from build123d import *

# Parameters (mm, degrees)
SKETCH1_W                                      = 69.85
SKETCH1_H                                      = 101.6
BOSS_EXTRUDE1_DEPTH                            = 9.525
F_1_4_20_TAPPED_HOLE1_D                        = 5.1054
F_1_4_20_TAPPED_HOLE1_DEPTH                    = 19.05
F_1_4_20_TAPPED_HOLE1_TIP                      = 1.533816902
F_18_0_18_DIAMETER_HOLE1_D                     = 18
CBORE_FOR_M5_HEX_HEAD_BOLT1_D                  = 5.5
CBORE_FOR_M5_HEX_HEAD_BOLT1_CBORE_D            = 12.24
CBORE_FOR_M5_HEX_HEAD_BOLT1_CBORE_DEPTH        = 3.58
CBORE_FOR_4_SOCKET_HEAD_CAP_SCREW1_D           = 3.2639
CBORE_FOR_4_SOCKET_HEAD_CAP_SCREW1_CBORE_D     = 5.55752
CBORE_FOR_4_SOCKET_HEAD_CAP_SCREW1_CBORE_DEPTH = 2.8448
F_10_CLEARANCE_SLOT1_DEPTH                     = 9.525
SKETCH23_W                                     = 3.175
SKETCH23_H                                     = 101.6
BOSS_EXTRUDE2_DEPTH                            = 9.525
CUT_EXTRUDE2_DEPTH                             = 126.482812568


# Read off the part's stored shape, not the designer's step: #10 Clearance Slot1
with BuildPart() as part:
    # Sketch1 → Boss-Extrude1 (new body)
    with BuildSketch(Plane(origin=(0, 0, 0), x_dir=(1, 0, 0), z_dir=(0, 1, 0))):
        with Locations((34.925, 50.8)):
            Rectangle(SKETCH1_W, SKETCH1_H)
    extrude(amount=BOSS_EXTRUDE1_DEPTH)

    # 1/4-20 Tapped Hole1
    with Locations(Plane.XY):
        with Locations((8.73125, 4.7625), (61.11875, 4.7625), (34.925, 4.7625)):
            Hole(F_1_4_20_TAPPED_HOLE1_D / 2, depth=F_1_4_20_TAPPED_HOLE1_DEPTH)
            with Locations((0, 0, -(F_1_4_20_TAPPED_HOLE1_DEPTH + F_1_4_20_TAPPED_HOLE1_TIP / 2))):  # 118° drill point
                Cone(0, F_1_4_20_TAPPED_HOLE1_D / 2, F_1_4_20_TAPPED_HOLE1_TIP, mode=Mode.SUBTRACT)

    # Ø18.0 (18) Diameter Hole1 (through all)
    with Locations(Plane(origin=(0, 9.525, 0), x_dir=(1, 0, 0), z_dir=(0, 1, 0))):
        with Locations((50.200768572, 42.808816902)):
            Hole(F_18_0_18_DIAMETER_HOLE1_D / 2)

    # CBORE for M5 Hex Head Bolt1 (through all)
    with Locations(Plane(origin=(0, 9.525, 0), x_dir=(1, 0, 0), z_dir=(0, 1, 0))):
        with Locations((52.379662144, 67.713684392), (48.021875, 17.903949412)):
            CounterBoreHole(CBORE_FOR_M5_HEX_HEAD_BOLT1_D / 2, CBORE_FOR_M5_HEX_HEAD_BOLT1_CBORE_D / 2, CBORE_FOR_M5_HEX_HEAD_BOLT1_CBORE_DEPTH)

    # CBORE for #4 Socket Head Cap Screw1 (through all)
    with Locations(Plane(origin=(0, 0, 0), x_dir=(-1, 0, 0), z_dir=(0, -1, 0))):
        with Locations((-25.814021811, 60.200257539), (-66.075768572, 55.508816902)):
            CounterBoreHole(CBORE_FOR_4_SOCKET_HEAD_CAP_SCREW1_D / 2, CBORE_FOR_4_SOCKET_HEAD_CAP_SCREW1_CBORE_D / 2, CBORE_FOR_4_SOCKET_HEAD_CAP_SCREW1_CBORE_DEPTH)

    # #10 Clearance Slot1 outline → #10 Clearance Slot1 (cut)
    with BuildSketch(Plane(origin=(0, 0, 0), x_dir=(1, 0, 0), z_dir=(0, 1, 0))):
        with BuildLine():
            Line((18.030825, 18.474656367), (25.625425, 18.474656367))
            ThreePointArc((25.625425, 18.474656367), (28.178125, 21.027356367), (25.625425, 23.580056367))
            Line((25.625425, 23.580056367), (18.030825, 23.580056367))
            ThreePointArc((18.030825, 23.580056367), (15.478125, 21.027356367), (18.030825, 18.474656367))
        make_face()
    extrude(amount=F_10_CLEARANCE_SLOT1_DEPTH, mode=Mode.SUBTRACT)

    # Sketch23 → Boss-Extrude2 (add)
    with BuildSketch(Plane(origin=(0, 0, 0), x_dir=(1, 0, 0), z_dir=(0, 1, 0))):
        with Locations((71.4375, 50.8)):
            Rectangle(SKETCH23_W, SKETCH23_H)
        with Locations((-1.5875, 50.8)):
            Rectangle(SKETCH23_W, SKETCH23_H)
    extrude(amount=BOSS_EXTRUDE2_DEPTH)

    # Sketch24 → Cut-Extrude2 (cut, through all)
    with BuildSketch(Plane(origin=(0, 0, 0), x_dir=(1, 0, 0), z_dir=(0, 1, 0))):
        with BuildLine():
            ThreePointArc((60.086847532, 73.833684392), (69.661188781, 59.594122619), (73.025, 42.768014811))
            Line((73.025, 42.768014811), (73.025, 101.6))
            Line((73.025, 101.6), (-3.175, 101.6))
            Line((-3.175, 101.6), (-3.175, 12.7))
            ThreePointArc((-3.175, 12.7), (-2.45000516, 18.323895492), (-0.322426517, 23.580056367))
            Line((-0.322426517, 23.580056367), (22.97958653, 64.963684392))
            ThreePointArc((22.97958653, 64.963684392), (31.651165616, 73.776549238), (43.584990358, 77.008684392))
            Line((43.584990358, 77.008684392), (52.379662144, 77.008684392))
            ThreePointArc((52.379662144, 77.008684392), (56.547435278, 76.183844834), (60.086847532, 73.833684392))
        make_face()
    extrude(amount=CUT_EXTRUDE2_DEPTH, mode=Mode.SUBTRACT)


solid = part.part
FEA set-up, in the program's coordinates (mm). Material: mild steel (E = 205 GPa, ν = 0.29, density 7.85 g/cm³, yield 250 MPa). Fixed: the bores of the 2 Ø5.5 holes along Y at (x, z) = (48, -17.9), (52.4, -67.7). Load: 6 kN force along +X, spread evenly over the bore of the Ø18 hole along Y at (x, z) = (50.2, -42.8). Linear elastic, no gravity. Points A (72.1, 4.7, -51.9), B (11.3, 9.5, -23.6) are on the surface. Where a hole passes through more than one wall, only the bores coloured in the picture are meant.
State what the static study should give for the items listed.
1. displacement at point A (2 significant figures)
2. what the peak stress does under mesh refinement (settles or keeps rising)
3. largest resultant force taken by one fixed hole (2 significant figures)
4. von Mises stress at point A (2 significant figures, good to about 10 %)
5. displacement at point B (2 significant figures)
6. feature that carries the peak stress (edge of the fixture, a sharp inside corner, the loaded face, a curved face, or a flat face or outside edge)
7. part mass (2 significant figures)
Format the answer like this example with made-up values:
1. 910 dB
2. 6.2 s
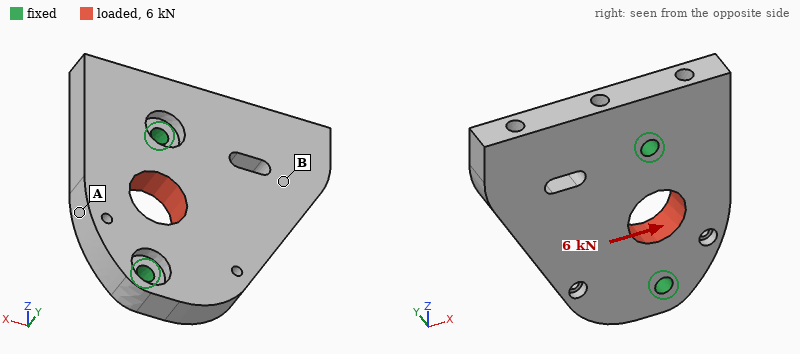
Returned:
1. 5.1 µm
2. keeps rising
3. 3.0 kN
4. 20 MPa
5. 7.5 µm
6. edge of the fixture
7. 310 g
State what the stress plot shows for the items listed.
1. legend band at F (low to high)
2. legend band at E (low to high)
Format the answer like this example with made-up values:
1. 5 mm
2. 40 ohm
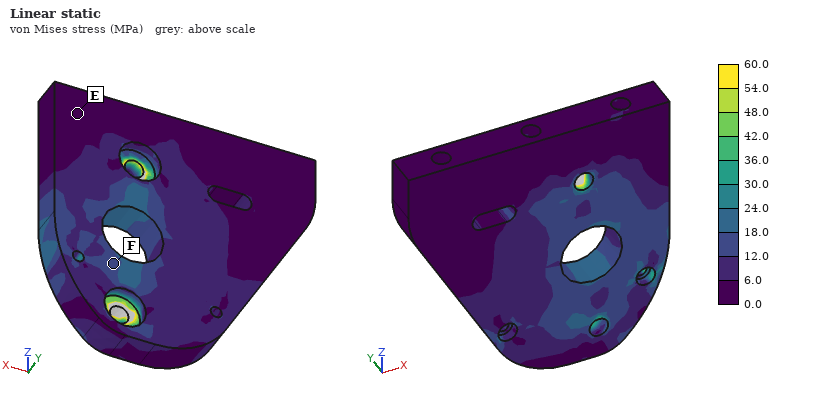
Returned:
1. 12.0 to 18.0 MPa
2. 0.0 to 6.0 MPa
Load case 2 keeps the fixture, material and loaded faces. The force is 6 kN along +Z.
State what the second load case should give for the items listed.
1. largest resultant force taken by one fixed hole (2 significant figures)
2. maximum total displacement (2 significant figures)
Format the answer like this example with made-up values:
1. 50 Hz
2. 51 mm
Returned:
1. 3.1 kN
2. 2.3 µm
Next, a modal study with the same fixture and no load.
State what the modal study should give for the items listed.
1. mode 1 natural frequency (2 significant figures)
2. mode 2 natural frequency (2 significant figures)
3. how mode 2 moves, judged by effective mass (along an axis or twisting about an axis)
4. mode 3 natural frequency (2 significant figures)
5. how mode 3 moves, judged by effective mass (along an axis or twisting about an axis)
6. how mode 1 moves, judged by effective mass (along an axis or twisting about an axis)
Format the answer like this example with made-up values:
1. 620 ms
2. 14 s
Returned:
1. 2400 Hz
2. 6000 Hz
3. twisting about X
4. 7800 Hz
5. along Y
6. along Y
